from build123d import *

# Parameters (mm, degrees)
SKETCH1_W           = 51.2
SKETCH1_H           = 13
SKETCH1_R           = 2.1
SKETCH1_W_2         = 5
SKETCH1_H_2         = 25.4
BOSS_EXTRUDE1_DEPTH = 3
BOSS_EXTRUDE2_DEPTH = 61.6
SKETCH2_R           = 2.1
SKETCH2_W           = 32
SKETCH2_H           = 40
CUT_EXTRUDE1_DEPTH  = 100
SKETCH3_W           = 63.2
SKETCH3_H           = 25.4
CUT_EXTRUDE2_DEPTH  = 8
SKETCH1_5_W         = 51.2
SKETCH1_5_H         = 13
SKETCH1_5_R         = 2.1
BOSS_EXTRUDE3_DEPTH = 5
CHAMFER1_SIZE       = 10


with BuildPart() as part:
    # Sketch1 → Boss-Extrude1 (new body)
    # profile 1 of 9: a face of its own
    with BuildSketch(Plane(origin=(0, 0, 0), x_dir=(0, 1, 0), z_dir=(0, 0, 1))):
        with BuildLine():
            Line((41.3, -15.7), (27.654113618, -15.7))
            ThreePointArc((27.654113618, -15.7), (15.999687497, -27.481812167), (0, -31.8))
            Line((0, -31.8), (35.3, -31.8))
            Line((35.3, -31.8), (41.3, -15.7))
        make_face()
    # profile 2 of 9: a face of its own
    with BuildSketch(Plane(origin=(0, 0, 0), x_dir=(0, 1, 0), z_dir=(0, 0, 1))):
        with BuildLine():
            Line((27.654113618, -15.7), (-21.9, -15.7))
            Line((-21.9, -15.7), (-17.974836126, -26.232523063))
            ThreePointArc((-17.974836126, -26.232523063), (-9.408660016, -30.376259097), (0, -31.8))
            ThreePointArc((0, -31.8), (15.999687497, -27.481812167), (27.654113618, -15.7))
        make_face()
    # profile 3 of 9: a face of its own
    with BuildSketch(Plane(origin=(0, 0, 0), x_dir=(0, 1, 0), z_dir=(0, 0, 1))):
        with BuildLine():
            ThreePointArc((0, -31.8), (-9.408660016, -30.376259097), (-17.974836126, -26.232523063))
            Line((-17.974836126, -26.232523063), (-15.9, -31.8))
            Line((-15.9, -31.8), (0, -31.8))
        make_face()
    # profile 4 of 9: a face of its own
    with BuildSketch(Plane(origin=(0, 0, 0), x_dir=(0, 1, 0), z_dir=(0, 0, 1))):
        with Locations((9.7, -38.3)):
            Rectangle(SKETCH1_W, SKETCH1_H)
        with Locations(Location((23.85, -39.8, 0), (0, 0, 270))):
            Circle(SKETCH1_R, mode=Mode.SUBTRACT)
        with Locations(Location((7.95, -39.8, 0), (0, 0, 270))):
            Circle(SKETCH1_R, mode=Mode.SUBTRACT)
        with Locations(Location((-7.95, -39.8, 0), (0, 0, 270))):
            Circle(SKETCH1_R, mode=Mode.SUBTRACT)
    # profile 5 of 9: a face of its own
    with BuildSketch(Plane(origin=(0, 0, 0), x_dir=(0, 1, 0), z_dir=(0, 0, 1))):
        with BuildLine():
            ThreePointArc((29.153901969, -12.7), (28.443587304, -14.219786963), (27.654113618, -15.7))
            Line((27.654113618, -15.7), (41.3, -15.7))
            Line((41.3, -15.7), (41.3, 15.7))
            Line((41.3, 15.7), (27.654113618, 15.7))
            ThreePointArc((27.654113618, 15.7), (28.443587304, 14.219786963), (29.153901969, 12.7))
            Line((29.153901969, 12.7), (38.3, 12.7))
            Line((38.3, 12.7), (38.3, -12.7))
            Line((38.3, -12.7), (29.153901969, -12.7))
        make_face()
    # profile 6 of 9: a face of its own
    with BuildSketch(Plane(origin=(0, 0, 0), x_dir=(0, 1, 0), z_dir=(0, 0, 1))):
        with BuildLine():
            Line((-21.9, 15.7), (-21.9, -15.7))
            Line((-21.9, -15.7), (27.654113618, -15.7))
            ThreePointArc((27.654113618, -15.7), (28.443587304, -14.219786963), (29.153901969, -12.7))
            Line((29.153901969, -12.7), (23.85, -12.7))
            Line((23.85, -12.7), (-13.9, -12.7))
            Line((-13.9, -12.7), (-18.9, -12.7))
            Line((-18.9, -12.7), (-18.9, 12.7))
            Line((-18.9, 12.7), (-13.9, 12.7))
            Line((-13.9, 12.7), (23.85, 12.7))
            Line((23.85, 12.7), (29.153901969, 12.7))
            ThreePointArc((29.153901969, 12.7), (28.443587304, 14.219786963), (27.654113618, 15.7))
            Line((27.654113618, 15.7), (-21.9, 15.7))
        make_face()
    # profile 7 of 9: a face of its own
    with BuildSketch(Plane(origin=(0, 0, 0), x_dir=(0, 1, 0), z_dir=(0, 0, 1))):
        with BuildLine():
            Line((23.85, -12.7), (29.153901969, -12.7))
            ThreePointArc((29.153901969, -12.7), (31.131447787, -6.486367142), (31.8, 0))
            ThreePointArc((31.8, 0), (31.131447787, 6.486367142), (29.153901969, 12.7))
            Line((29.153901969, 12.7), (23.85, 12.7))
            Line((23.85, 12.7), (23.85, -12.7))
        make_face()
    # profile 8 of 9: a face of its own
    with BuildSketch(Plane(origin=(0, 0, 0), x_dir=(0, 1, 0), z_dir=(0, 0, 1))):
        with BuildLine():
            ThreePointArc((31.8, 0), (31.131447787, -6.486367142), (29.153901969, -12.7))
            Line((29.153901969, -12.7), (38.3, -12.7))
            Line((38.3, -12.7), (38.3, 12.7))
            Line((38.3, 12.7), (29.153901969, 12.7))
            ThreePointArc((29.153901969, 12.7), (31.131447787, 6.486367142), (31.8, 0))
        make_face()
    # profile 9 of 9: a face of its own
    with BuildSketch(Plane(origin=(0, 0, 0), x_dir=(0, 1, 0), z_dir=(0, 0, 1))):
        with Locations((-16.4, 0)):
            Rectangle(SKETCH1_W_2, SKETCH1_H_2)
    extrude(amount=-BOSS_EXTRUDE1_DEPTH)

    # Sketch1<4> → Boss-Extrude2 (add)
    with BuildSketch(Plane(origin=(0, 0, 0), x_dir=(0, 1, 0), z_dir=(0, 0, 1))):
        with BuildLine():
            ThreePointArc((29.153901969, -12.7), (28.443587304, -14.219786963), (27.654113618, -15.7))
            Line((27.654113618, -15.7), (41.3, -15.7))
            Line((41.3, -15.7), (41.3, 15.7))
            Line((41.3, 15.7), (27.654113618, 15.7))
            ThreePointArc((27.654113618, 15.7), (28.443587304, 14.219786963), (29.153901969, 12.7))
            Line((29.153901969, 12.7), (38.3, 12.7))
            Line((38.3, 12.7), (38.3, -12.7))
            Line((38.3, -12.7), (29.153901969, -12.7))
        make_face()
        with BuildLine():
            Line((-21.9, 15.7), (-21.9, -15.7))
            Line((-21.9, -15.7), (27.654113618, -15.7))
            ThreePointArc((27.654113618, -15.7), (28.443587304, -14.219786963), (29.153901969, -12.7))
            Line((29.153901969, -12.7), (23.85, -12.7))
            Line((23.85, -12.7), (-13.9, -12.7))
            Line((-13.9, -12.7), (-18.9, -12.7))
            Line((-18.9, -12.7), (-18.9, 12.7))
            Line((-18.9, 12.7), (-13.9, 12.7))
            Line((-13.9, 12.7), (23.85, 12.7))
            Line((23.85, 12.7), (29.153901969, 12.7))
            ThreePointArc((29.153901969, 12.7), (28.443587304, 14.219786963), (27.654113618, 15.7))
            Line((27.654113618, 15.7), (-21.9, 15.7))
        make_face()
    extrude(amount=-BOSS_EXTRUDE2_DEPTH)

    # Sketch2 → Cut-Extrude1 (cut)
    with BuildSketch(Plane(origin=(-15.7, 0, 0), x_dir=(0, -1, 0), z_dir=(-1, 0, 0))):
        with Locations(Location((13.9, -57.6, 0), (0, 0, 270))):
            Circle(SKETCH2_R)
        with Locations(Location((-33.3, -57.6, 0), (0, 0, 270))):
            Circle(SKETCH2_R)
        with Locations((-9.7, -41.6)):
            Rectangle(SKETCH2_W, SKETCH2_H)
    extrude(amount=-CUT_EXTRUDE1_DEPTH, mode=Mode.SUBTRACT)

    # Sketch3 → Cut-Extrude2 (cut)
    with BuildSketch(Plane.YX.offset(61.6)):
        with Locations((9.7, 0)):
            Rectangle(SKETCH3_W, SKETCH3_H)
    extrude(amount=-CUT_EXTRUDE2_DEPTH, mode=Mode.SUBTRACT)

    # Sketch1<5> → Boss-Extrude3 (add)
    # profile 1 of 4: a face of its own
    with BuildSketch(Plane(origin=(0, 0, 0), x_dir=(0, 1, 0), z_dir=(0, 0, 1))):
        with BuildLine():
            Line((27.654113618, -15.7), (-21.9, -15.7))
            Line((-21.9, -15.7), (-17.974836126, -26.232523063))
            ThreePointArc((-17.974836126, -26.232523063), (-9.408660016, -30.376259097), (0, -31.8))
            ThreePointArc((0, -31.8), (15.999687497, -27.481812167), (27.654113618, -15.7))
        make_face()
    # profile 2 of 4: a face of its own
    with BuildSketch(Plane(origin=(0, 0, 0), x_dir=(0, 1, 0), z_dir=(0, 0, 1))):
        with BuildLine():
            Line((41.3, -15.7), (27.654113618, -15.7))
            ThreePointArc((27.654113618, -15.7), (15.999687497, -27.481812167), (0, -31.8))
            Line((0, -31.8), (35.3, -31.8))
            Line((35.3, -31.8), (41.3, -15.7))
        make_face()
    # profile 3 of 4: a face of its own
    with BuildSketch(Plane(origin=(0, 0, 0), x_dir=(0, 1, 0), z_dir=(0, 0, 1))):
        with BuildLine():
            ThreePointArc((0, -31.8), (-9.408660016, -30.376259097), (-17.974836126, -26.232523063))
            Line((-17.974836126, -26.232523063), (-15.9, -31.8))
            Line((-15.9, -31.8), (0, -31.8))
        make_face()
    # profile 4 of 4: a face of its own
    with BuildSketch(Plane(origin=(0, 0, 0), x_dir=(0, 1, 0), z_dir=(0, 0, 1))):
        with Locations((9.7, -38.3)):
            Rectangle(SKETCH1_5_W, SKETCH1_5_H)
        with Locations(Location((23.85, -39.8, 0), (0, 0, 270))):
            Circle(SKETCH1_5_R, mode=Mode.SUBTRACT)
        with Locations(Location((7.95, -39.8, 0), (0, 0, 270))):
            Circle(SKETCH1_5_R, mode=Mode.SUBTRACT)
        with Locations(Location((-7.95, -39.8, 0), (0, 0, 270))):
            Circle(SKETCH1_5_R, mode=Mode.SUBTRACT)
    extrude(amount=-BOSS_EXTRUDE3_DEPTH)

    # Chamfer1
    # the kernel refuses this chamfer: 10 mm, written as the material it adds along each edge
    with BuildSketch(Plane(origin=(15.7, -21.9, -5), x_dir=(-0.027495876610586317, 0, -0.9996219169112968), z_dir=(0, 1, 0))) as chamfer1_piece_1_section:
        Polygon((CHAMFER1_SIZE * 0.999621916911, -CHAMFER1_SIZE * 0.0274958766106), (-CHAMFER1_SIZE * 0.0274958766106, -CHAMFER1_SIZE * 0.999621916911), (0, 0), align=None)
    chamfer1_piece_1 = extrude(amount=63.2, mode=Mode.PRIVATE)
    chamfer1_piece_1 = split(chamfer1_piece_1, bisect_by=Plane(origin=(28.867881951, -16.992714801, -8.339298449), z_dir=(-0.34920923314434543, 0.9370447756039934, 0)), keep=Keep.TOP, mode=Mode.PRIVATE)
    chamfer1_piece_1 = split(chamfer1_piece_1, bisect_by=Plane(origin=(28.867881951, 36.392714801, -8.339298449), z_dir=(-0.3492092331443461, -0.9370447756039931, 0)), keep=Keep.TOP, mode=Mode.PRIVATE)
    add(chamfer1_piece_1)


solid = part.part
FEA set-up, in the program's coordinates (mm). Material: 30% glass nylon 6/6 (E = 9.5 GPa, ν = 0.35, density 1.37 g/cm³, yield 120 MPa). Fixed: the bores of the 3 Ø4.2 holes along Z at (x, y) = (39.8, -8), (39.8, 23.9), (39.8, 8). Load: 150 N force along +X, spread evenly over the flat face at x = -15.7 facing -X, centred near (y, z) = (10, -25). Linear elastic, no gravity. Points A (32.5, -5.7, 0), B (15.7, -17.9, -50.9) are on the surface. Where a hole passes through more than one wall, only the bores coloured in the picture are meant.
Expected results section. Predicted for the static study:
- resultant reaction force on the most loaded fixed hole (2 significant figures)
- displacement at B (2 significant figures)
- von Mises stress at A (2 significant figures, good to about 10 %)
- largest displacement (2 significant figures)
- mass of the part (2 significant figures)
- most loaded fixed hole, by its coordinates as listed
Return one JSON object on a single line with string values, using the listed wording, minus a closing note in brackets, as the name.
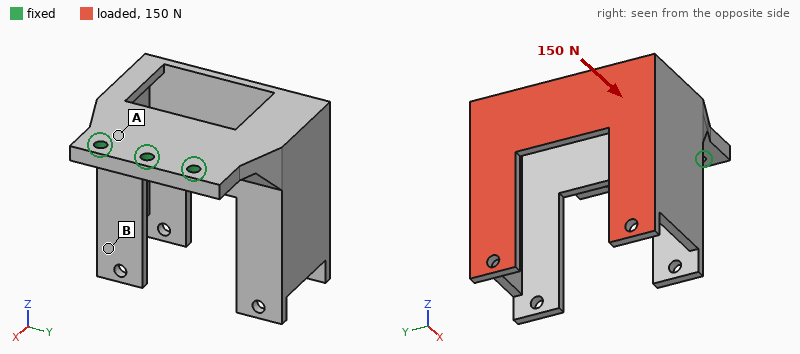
{"resultant reaction force on the most loaded fixed hole": "73 N", "displacement at B": "0.64 mm", "von Mises stress at A": "14 MPa", "largest displacement": "1.0 mm", "mass of the part": "49 g", "most loaded fixed hole, by its coordinates as listed": "(39.8, 23.9)"}
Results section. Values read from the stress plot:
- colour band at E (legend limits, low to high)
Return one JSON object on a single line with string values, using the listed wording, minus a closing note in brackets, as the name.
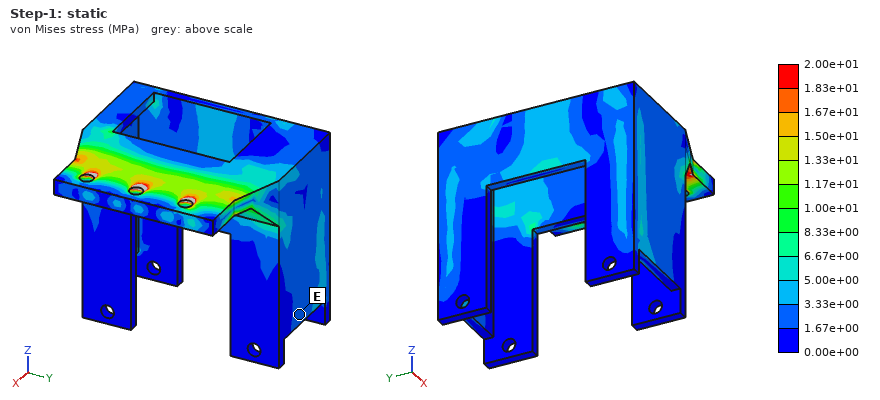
{"colour band at E": "1.67e+00 to 3.33e+00 MPa"}
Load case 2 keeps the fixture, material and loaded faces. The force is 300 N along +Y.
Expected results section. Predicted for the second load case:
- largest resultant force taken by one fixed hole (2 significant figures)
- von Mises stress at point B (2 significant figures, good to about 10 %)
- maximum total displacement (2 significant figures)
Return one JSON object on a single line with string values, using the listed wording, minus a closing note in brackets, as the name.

{"largest resultant force taken by one fixed hole": "540 N", "von Mises stress at point B": "4.5 MPa", "maximum total displacement": "1.3 mm"}
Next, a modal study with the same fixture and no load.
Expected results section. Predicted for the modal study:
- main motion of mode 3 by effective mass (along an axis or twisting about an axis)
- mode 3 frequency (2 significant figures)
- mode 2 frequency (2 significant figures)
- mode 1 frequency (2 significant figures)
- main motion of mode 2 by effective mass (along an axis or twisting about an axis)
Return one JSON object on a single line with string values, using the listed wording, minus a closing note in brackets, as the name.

{"main motion of mode 3 by effective mass": "along Y", "mode 3 frequency": "1300 Hz", "mode 2 frequency": "560 Hz", "mode 1 frequency": "330 Hz", "main motion of mode 2 by effective mass": "along Y"}
